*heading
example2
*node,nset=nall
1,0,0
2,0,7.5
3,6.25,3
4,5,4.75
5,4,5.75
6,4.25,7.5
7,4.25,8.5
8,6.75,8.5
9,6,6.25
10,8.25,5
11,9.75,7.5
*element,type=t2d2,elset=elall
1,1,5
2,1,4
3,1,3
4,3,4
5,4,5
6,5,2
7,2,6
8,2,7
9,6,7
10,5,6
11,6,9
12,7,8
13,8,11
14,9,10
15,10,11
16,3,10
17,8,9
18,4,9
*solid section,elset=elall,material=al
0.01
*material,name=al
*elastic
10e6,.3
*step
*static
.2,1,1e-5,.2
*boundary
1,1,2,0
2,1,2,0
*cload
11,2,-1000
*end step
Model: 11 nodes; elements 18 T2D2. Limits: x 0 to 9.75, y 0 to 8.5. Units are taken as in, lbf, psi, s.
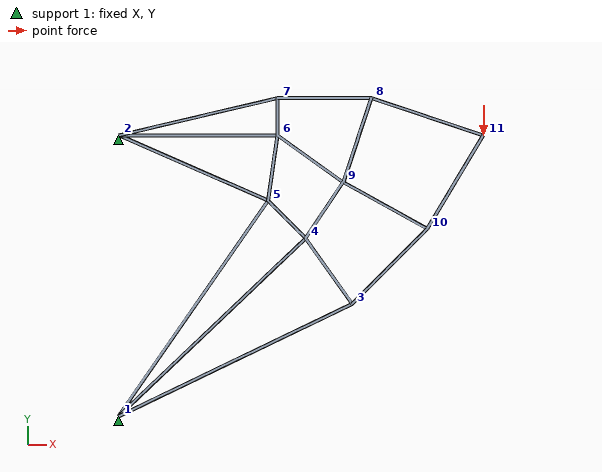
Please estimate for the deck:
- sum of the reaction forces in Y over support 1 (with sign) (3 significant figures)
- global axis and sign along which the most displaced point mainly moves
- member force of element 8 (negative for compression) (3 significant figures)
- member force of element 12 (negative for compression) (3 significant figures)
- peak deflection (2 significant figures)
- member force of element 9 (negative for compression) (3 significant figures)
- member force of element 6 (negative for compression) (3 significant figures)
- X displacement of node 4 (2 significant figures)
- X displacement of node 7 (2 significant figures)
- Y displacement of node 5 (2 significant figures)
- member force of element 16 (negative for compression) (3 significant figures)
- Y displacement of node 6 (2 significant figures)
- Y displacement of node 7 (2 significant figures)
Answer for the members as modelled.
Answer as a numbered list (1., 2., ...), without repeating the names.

1. 1000 lbf
2. -Y
3. 571 lbf
4. 556 lbf
5. 0.20 in
6. -131 lbf
7. 508 lbf
8. 0.017 in
9. 0.037 in
10. -0.041 in
11. -1010 lbf
12. -0.048 in
13. -0.049 in
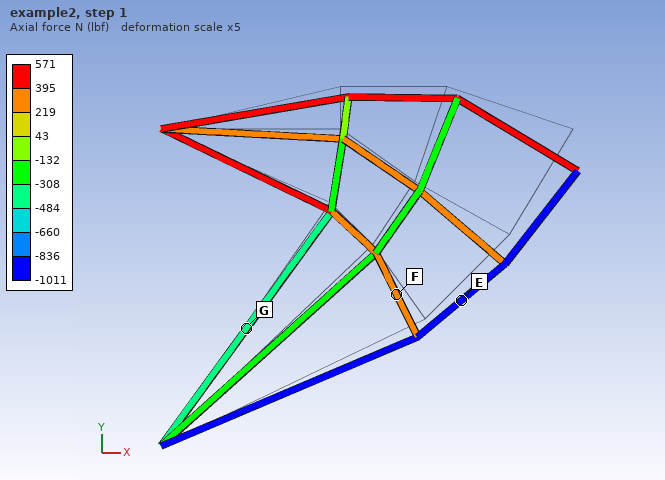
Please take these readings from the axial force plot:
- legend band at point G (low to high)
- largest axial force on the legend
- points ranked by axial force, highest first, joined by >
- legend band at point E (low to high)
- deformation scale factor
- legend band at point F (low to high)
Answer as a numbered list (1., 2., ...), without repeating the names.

1. -484 to -308 lbf
2. 571 lbf
3. F > G > E
4. -1011 to -836 lbf
5. 5
6. 219 to 395 lbf
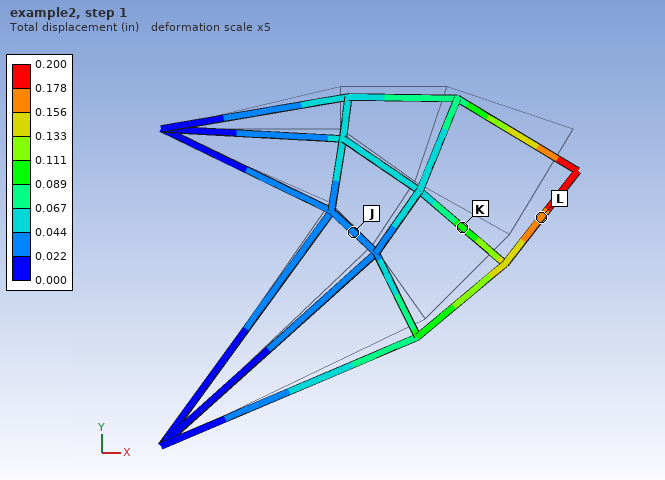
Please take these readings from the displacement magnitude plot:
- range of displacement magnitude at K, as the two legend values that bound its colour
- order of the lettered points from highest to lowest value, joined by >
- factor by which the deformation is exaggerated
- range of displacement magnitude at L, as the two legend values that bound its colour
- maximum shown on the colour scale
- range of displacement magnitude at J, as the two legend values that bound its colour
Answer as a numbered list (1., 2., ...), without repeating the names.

1. 0.089 to 0.111 in
2. L > K > J
3. 5
4. 0.156 to 0.178 in
5. 0.200 in
6. 0.022 to 0.044 in
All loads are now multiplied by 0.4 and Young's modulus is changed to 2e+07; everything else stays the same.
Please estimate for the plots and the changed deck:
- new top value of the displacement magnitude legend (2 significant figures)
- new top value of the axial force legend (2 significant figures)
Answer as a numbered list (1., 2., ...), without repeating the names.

1. 0.040 in
2. 230 lbf
